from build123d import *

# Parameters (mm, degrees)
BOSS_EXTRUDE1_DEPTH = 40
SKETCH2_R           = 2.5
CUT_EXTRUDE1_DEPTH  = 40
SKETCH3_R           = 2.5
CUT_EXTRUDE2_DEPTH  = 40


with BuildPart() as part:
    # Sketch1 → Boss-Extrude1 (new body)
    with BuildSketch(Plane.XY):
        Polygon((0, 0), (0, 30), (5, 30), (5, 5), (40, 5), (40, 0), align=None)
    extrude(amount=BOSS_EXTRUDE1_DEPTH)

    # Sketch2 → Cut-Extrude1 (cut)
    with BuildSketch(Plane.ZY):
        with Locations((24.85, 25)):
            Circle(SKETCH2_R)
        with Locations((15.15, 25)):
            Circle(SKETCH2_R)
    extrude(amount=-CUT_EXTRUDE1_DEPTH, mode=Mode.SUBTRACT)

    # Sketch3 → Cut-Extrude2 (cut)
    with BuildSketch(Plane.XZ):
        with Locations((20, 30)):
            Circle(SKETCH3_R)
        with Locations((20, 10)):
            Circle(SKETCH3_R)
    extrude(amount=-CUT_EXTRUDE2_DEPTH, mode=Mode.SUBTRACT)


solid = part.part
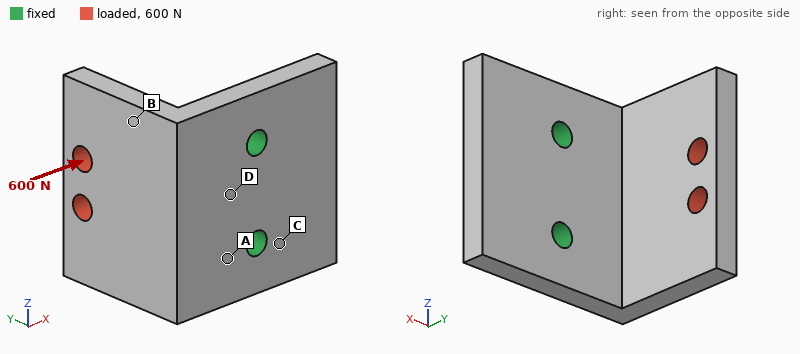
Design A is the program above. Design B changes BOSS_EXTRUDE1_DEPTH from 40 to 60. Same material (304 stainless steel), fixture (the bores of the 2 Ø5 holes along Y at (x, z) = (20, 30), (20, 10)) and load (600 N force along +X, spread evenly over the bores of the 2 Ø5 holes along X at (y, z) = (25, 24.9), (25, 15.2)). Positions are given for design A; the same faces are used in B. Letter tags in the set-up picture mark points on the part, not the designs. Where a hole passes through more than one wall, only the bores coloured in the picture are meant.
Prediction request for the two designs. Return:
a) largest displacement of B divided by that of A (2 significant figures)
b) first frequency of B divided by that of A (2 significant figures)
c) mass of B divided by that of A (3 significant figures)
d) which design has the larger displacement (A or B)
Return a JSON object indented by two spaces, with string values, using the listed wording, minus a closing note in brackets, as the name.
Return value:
{
  "largest displacement of B divided by that of A": "0.81",
  "first frequency of B divided by that of A": "0.86",
  "mass of B divided by that of A": "1.52",
  "which design has the larger displacement": "A"
}
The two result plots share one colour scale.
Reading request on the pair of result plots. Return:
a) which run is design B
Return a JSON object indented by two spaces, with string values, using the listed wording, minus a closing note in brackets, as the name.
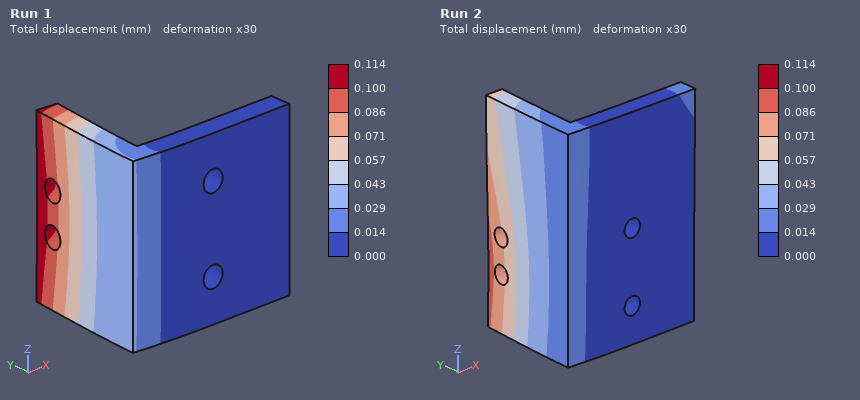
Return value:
{
  "which run is design B": "Run 2"
}
